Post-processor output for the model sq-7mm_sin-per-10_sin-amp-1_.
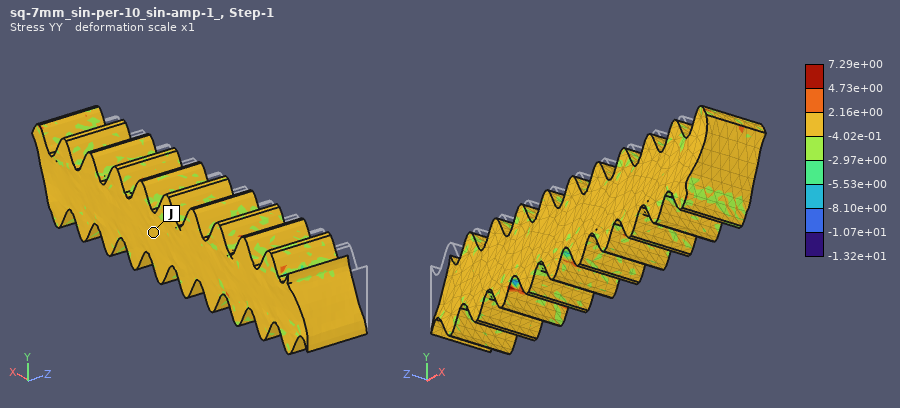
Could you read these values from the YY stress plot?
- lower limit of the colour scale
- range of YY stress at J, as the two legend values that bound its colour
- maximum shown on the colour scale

-1.32e+01
-4.02e-01 to 2.16e+00
7.29e+00
